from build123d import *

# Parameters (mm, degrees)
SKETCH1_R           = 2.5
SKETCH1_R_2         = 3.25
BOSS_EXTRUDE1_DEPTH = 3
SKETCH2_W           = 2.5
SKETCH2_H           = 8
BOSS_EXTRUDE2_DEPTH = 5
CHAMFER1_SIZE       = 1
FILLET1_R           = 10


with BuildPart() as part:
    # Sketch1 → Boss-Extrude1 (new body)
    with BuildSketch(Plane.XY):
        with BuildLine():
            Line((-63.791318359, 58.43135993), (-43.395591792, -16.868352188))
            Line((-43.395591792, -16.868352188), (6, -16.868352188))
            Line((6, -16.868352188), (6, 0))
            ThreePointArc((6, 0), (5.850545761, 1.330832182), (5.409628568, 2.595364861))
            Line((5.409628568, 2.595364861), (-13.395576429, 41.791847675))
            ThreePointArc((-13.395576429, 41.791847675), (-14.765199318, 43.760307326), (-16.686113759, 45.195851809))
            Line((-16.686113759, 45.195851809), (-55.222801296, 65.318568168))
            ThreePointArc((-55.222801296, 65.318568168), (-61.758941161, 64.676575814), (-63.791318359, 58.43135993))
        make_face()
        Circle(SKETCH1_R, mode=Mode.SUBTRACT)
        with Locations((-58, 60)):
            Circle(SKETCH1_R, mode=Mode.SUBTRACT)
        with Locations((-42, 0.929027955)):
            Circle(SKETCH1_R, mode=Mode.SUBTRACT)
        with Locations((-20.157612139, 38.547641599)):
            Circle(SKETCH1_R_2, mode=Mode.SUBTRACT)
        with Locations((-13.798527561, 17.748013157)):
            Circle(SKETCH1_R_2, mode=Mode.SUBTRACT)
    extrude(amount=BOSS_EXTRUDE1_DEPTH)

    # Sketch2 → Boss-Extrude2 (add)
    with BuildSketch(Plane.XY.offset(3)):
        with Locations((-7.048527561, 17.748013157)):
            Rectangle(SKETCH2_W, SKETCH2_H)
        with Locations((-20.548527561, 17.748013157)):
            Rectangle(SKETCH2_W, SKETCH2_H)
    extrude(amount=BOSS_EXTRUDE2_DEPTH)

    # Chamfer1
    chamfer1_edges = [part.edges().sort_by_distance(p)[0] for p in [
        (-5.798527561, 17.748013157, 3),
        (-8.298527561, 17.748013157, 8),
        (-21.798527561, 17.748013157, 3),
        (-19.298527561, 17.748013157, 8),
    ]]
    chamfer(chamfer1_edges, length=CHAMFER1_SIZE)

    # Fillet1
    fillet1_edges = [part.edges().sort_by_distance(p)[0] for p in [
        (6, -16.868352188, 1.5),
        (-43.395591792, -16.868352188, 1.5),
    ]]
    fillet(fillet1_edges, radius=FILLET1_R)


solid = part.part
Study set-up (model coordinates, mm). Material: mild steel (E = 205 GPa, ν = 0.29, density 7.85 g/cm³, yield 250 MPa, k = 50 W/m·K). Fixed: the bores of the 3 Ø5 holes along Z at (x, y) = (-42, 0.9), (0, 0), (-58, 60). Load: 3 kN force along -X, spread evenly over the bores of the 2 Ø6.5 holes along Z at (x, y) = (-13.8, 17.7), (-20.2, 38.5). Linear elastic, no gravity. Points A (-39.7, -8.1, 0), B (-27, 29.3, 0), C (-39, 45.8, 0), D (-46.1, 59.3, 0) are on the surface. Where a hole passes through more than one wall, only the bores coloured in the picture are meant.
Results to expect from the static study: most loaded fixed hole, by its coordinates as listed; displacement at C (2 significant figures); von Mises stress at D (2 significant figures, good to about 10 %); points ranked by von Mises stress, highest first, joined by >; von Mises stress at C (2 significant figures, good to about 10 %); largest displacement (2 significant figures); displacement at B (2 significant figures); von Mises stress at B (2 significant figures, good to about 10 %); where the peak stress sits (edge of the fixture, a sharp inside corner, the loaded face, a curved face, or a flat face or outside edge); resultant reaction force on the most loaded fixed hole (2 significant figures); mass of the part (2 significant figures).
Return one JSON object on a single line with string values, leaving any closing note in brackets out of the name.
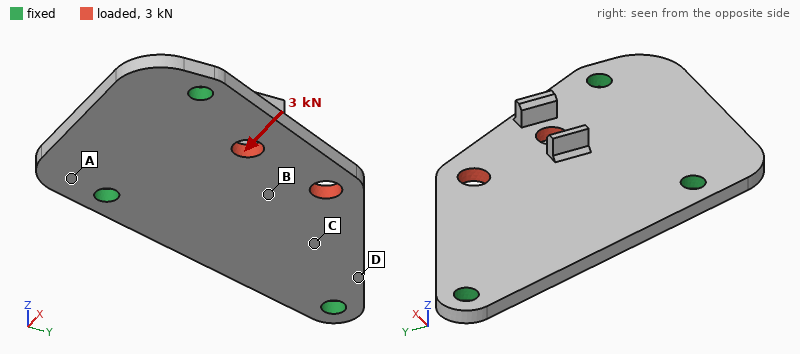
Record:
{"most loaded fixed hole, by its coordinates as listed": "(-42, 0.9)", "displacement at C": "4.4 µm", "von Mises stress at D": "28 MPa", "points ranked by von Mises stress, highest first, joined by >": "D > C > B > A", "von Mises stress at C": "20 MPa", "largest displacement": "7.3 µm", "displacement at B": "5.2 µm", "von Mises stress at B": "14 MPa", "where the peak stress sits": "edge of the fixture", "resultant reaction force on the most loaded fixed hole": "1.5 kN", "mass of the part": "84 g"}
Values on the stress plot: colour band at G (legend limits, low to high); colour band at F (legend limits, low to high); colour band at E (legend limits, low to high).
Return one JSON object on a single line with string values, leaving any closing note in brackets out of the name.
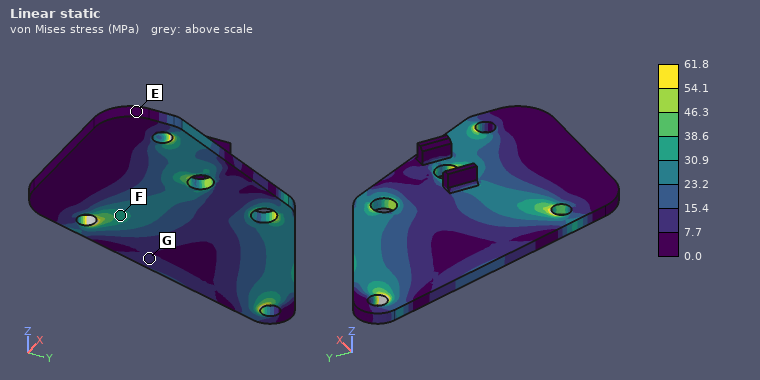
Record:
{"colour band at G": "7.7 to 15.4 MPa", "colour band at F": "30.9 to 38.6 MPa", "colour band at E": "0.0 to 7.7 MPa"}
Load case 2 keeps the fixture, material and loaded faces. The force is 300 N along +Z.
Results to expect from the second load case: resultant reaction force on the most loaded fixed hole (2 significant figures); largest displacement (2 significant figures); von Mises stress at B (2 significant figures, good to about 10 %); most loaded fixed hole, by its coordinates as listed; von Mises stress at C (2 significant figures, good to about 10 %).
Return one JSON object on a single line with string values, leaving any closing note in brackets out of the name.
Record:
{"resultant reaction force on the most loaded fixed hole": "170 N", "largest displacement": "96 µm", "von Mises stress at B": "34 MPa", "most loaded fixed hole, by its coordinates as listed": "(0, 0)", "von Mises stress at C": "28 MPa"}
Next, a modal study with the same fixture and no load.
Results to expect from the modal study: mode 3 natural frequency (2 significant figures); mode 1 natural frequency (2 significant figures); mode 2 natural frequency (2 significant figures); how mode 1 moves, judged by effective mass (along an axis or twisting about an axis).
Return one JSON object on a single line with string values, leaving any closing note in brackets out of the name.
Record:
{"mode 3 natural frequency": "6400 Hz", "mode 1 natural frequency": "2400 Hz", "mode 2 natural frequency": "5100 Hz", "how mode 1 moves, judged by effective mass": "along Z"}
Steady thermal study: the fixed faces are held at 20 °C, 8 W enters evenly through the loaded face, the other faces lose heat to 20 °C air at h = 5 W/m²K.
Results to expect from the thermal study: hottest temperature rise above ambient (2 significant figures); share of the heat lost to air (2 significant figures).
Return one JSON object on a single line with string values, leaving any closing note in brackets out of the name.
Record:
{"hottest temperature rise above ambient": "34 K", "share of the heat lost to air": "5.5 %"}
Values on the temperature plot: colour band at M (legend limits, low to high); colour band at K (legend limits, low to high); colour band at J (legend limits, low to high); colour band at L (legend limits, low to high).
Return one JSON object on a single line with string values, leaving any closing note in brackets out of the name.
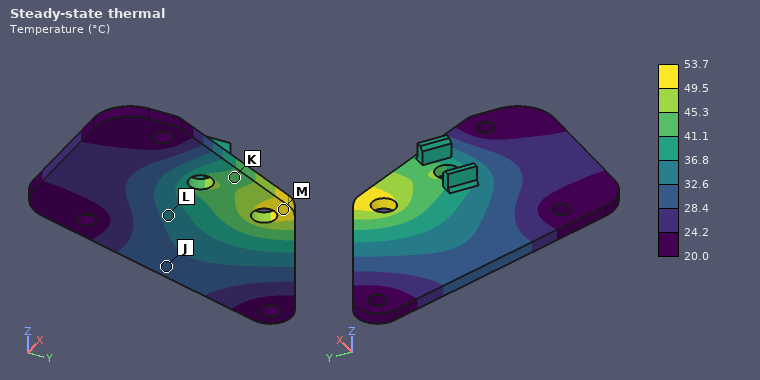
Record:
{"colour band at M": "49.5 to 53.7 °C", "colour band at K": "41.1 to 45.3 °C", "colour band at J": "28.4 to 32.6 °C", "colour band at L": "32.6 to 36.8 °C"}
